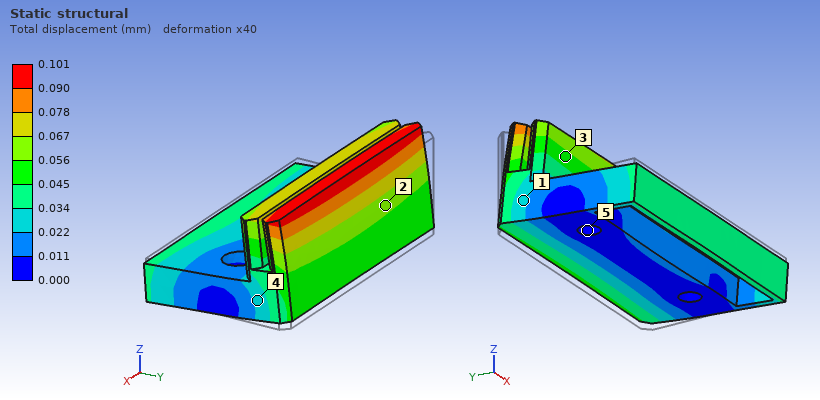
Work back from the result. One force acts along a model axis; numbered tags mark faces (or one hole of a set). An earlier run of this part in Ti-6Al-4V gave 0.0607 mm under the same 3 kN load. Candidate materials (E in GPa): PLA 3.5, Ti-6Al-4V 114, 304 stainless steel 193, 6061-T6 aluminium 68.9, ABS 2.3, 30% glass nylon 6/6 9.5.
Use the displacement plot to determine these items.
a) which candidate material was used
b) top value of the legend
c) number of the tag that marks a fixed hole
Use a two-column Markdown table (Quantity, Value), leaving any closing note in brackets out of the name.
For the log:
| Quantity | Value |
|---|---|
| which candidate material was used | 6061-T6 aluminium |
| top value of the legend | 0.101 mm |
| number of the tag that marks a fixed hole | 5 |
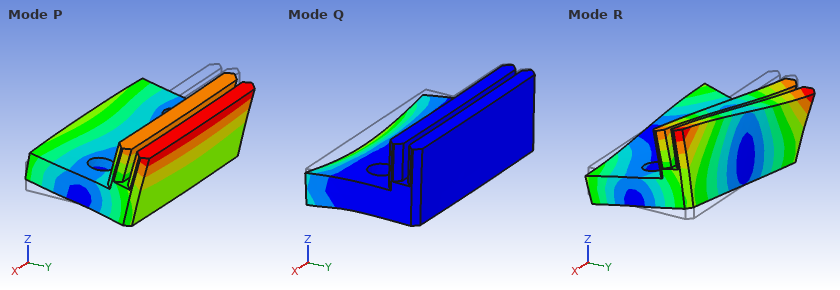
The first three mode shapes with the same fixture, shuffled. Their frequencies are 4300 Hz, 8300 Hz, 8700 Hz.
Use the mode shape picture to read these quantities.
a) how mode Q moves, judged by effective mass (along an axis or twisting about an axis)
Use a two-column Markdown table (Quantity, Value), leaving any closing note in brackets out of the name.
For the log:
| Quantity | Value |
|---|---|
| how mode Q moves, judged by effective mass | along Z |
